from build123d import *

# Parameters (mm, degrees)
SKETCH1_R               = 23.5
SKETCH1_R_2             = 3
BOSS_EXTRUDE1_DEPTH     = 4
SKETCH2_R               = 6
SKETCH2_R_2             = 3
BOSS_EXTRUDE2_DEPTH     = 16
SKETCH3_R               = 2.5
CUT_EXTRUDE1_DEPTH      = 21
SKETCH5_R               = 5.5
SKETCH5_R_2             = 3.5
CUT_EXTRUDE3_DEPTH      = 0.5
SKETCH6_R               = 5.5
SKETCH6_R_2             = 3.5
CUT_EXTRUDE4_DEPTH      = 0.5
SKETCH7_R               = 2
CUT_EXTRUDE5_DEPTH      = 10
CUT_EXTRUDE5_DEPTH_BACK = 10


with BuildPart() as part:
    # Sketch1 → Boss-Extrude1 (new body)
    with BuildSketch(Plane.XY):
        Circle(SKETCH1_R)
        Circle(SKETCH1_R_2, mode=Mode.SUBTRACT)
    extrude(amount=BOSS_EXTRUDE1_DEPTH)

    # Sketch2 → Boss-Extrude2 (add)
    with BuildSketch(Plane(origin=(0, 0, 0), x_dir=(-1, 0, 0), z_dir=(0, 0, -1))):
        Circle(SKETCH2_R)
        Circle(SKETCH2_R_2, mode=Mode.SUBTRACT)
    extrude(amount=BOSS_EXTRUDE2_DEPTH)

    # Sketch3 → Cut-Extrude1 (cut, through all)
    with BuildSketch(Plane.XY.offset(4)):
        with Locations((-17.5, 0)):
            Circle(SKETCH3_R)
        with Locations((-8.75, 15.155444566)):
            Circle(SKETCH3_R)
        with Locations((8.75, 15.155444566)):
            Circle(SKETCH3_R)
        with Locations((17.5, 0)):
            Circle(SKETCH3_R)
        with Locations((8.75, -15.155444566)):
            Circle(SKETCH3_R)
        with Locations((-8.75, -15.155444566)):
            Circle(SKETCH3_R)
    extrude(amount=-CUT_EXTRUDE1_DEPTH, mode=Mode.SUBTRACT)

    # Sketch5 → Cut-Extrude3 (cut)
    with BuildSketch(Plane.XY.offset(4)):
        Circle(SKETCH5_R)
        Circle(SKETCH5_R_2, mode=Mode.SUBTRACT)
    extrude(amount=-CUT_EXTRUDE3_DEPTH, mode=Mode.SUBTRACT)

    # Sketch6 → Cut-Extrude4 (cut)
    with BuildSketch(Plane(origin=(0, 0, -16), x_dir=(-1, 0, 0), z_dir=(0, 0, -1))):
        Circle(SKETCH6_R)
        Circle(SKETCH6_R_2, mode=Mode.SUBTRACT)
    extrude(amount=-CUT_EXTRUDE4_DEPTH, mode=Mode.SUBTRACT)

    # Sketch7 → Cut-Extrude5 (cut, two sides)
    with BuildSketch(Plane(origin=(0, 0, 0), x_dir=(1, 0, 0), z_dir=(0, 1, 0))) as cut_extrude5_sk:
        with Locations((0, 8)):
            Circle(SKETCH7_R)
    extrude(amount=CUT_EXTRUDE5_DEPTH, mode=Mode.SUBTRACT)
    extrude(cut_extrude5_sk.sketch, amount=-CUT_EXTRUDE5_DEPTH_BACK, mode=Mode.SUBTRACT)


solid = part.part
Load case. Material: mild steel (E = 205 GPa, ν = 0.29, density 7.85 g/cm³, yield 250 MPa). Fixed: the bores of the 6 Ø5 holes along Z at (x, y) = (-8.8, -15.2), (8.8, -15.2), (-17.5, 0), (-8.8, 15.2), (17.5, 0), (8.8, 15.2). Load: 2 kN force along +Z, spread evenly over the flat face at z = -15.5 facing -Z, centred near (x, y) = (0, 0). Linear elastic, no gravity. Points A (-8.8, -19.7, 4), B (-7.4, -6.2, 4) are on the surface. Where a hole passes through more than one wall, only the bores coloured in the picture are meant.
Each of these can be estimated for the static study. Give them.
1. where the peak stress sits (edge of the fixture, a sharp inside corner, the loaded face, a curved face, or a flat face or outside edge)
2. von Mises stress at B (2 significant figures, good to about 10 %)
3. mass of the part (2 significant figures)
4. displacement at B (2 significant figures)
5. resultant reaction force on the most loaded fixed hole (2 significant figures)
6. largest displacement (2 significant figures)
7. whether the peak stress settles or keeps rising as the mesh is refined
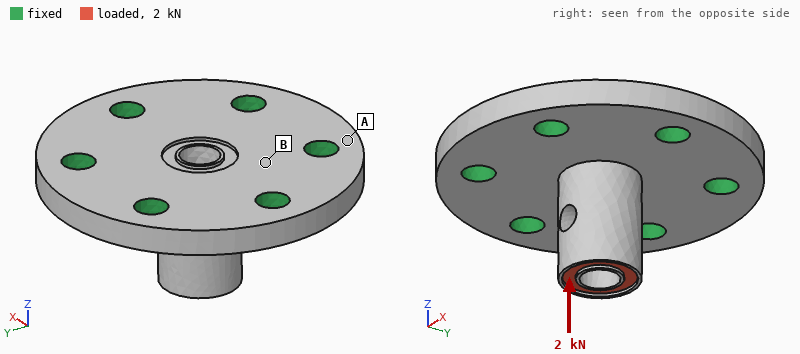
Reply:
edge of the fixture
27 MPa
59 g
3.2 µm
370 N
8.1 µm
keeps rising
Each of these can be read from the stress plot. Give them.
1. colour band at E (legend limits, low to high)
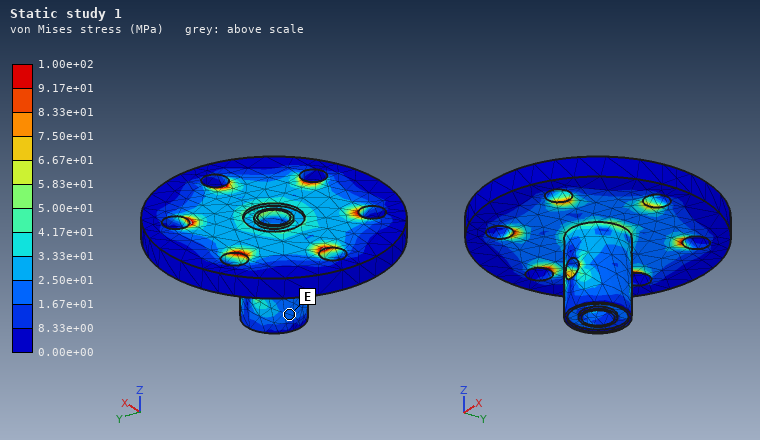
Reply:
1.67e+01 to 2.50e+01 MPa
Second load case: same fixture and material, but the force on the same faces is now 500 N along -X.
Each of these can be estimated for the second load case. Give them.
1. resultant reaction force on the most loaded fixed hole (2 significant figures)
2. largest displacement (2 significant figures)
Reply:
280 N
15 µm
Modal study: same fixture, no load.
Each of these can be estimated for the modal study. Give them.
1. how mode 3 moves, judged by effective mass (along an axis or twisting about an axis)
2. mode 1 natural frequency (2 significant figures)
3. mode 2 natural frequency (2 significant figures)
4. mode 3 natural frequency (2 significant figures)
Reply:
along Z
16 kHz
16 kHz
23 kHz
